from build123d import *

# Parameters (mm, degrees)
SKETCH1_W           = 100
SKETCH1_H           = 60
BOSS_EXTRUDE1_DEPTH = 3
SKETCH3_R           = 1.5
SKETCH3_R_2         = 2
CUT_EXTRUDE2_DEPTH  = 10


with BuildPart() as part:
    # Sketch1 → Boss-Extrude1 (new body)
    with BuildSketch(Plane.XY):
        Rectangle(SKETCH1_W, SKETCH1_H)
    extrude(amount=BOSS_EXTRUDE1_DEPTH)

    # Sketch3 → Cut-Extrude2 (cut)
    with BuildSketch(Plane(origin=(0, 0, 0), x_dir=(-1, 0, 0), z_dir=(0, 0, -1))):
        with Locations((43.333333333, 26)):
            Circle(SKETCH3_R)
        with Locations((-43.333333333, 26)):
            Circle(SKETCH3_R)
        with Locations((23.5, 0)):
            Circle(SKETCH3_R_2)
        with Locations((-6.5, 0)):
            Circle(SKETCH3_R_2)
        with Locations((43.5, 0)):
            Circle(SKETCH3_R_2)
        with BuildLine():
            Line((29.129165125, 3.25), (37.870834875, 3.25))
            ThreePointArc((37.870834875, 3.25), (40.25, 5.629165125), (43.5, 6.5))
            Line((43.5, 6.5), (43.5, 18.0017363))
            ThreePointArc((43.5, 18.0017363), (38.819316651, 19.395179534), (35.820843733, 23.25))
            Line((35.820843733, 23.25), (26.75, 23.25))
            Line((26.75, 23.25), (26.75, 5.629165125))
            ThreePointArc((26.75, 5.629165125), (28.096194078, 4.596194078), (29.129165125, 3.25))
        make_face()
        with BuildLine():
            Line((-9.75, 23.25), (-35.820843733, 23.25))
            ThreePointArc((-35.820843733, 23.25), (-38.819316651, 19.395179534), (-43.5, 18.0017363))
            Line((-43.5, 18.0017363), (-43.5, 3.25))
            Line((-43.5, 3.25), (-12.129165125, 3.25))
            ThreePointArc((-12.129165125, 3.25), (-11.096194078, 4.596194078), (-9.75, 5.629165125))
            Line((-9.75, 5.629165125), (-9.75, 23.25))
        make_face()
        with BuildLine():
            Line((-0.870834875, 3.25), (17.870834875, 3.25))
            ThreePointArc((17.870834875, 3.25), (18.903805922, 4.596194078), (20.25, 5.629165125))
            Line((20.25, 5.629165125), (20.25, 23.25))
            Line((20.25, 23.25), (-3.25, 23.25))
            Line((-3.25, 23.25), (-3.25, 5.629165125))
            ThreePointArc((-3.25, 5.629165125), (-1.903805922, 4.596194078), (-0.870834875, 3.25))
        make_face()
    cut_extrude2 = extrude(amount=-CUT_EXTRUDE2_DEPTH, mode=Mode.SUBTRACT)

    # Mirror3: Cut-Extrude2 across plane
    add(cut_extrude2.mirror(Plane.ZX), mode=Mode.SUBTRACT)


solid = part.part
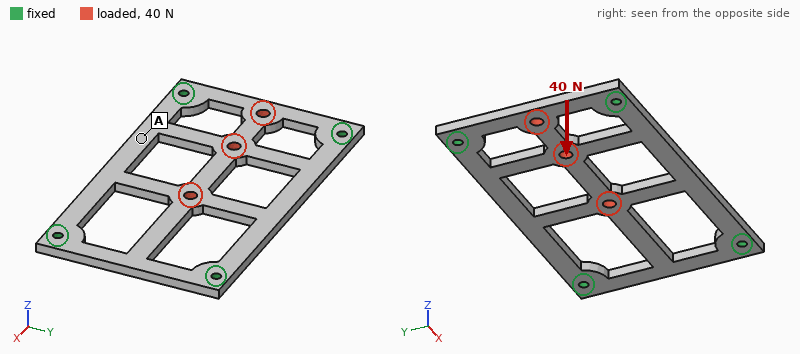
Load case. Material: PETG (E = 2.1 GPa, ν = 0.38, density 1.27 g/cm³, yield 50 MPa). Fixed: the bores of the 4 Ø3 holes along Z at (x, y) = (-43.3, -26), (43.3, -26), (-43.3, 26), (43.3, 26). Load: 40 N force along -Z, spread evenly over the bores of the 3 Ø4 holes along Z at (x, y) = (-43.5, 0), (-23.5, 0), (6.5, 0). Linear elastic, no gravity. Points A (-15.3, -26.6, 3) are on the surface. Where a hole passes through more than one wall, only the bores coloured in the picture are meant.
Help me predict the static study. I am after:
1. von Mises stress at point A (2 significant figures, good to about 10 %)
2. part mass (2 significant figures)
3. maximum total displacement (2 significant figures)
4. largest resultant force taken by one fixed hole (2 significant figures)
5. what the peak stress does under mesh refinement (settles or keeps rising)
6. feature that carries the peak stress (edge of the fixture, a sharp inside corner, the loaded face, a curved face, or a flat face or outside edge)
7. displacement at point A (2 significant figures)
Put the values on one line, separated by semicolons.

2.7 MPa; 12 g; 1.1 mm; 15 N; keeps rising; edge of the fixture; 0.47 mm
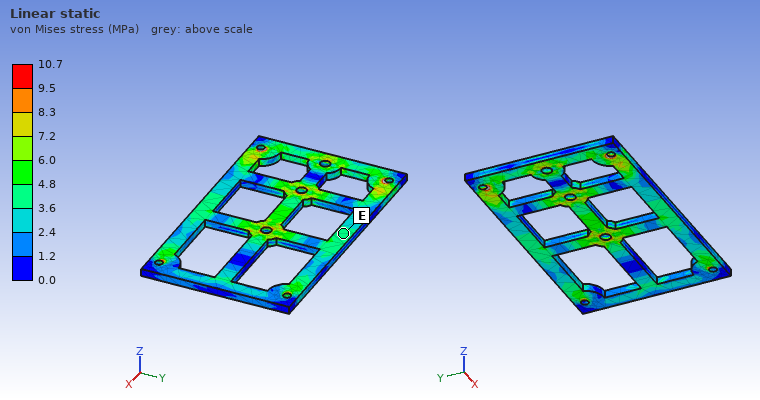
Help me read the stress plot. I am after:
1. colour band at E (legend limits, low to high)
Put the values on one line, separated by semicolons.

3.6 to 4.8 MPa
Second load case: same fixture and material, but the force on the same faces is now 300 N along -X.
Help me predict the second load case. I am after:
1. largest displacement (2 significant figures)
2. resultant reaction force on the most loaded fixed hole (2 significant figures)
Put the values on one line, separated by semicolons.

0.33 mm; 93 N
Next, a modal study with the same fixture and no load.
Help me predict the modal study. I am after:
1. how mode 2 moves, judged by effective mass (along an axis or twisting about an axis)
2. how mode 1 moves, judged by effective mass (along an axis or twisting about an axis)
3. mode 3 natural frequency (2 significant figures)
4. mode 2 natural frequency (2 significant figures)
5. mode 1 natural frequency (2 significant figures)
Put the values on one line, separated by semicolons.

twisting about X; along Z; 950 Hz; 630 Hz; 420 Hz
